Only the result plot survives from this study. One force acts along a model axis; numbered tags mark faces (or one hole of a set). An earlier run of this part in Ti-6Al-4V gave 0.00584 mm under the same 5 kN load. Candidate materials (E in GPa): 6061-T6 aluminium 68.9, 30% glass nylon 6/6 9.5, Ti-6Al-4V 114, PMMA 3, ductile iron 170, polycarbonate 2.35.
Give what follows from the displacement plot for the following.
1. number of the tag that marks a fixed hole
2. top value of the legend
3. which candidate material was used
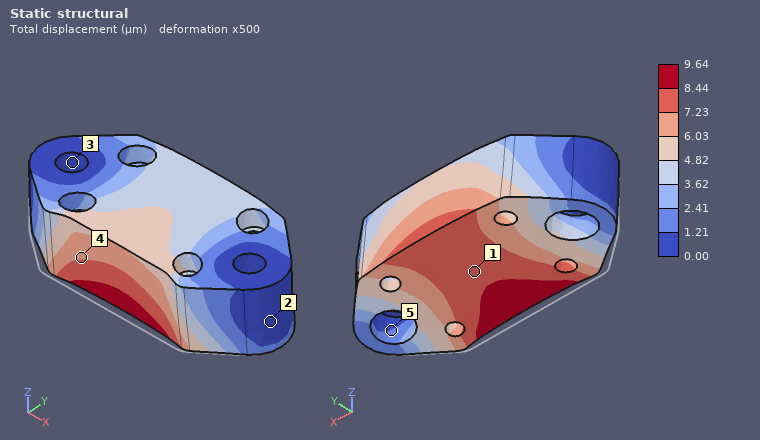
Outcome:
3
9.64 µm
6061-T6 aluminium
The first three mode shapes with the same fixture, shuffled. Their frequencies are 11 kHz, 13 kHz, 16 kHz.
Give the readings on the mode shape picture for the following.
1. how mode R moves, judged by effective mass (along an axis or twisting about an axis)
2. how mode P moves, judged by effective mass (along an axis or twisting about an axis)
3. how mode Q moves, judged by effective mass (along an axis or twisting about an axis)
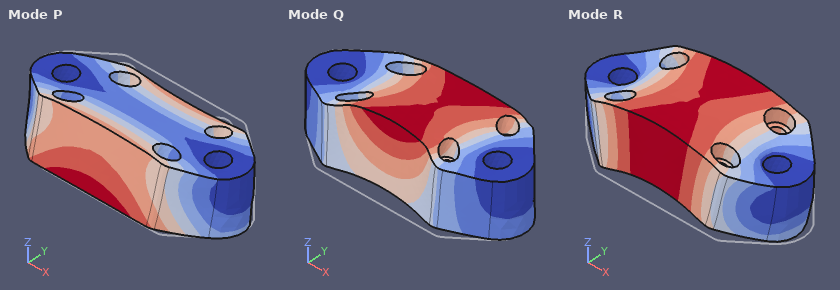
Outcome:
along Z
along Y
along Y
